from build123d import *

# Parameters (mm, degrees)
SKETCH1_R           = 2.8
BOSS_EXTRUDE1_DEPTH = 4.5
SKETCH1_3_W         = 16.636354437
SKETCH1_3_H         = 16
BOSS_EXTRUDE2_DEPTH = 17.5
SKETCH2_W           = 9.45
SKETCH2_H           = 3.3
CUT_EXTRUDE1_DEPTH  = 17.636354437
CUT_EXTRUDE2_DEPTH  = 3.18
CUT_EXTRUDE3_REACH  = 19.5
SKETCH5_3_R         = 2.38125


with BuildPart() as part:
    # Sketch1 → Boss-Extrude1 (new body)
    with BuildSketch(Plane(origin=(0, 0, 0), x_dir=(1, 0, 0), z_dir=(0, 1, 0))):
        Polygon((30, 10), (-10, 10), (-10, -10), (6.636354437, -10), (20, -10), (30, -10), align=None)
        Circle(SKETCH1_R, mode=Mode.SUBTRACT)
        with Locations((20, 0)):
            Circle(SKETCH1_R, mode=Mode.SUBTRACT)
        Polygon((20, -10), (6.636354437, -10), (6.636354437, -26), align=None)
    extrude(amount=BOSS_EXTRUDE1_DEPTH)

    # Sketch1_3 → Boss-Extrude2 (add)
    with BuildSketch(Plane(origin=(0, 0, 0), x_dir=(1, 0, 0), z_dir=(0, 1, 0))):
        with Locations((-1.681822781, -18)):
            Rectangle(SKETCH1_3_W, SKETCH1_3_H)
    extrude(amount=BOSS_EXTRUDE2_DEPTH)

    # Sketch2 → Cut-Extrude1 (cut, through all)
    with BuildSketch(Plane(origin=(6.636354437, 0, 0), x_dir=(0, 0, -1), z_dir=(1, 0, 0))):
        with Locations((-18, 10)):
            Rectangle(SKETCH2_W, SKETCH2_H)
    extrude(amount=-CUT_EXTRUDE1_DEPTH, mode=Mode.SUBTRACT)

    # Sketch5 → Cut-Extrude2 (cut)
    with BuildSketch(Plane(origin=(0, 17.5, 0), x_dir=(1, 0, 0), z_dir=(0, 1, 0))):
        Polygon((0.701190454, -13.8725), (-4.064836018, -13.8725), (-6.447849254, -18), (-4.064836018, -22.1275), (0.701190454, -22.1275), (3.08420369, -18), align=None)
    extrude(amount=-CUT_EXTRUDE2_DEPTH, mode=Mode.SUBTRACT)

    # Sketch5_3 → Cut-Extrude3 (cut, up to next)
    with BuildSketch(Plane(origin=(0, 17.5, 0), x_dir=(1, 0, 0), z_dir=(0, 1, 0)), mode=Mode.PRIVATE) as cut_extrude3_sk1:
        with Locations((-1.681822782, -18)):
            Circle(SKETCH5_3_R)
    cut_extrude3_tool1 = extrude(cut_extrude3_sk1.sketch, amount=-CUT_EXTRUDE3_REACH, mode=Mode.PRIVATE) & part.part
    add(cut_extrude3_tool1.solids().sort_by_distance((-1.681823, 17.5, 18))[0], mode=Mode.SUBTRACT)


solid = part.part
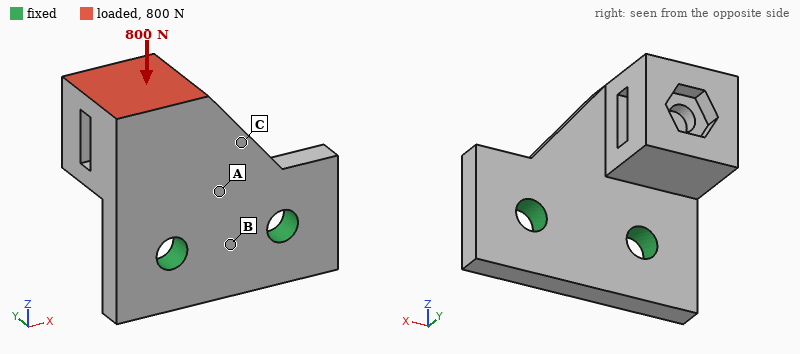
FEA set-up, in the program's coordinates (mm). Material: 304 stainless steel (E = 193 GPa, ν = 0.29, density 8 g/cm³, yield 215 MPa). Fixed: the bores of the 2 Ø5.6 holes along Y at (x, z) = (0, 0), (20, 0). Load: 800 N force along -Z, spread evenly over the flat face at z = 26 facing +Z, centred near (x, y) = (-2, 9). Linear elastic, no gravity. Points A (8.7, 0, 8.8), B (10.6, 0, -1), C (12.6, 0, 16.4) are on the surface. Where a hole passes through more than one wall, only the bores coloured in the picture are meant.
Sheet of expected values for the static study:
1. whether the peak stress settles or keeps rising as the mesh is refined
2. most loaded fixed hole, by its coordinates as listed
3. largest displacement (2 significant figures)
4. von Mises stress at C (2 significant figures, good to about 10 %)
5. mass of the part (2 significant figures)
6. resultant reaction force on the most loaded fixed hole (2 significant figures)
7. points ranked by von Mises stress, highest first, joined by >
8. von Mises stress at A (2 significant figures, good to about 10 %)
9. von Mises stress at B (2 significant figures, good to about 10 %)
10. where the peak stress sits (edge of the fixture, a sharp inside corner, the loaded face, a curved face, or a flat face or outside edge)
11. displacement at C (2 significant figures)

keeps rising
(0, 0)
39 µm
28 MPa
62 g
810 N
A > C > B
40 MPa
11 MPa
edge of the fixture
11 µm
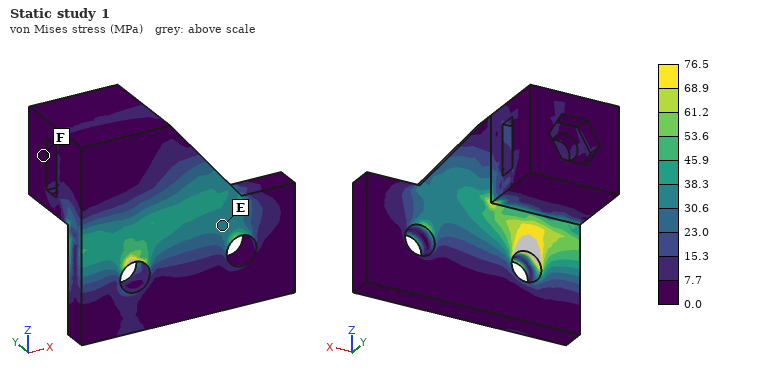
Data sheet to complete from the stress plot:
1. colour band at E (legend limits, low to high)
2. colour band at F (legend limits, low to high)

30.6 to 38.3 MPa
0.0 to 7.7 MPa
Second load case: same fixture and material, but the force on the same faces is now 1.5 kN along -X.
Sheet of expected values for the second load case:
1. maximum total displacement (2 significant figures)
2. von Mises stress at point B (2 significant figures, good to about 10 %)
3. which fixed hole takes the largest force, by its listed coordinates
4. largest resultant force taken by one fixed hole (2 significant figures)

35 µm
18 MPa
(20, 0)
1.9 kN
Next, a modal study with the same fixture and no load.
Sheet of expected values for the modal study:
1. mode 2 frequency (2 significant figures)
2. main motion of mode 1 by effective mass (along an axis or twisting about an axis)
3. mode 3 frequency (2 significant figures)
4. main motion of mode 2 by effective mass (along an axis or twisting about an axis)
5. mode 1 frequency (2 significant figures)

8100 Hz
along Y
16 kHz
along X
3400 Hz
